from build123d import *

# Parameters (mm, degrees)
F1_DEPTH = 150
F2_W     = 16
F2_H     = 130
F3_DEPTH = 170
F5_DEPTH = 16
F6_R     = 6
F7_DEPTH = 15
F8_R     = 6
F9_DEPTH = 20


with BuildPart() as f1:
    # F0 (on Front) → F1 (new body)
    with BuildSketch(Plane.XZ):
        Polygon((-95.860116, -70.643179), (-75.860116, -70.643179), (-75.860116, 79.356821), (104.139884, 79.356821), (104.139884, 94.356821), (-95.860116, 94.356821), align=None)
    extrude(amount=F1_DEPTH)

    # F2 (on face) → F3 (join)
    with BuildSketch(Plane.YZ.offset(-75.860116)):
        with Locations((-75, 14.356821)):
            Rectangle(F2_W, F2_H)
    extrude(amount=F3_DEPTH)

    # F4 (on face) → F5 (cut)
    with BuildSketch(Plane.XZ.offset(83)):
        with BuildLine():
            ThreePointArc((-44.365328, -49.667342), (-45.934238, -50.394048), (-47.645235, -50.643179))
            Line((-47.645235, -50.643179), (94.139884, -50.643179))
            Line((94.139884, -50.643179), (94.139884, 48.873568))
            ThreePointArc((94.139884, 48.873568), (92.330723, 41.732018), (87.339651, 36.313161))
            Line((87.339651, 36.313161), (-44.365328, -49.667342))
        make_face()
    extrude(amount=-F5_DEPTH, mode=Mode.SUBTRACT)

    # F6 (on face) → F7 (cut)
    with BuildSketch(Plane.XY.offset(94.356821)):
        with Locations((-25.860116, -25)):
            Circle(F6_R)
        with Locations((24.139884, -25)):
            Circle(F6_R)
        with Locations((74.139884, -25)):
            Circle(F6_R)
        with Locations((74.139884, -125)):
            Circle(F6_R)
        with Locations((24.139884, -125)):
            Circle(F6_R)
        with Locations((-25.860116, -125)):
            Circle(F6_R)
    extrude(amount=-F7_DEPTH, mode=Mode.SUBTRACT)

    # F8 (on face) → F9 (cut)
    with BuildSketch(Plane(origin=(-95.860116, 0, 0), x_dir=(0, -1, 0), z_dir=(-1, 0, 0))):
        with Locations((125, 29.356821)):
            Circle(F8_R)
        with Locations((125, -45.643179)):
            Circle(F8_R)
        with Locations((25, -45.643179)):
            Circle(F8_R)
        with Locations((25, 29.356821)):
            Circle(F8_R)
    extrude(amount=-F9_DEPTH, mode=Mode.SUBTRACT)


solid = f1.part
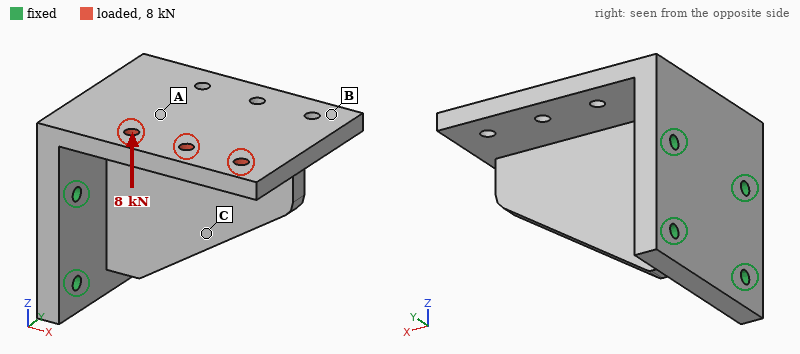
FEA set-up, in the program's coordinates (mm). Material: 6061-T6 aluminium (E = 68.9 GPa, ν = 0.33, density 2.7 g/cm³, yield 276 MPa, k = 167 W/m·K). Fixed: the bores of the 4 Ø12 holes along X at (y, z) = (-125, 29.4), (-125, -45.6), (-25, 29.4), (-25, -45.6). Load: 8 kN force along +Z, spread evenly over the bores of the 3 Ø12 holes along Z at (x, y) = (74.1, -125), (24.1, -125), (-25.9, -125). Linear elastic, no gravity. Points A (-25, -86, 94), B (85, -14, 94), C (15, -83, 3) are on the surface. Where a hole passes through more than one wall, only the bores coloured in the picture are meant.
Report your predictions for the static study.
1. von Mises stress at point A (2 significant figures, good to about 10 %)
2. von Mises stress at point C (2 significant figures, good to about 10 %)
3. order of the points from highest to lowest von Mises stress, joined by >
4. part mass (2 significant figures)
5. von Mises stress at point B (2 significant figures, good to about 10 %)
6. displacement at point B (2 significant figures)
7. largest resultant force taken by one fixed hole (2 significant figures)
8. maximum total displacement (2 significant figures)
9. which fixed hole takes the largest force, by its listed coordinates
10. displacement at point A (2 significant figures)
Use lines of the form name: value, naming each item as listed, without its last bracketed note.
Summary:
von Mises stress at point A: 35 MPa
von Mises stress at point C: 20 MPa
order of the points from highest to lowest von Mises stress, joined by >: A > C > B
part mass: 3.1 kg
von Mises stress at point B: 6.7 MPa
displacement at point B: 0.087 mm
largest resultant force taken by one fixed hole: 6.6 kN
maximum total displacement: 0.57 mm
which fixed hole takes the largest force, by its listed coordinates: (-125, 29.4)
displacement at point A: 0.097 mm
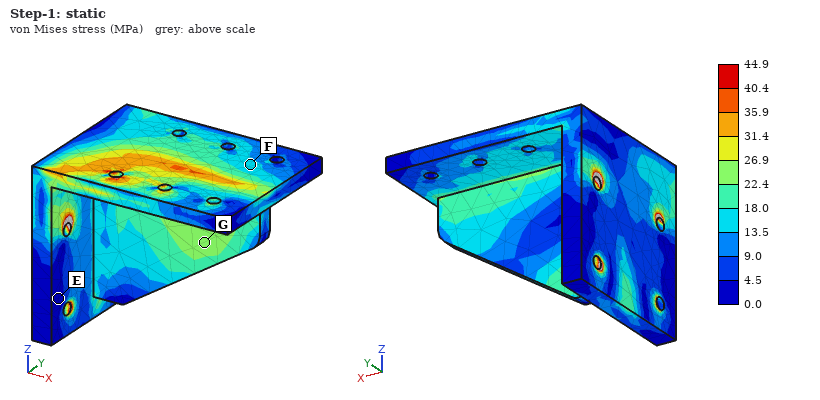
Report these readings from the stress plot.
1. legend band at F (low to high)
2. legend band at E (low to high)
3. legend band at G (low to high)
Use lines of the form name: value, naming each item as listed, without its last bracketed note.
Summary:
legend band at F: 13.5 to 18.0 MPa
legend band at E: 0.0 to 4.5 MPa
legend band at G: 22.4 to 26.9 MPa
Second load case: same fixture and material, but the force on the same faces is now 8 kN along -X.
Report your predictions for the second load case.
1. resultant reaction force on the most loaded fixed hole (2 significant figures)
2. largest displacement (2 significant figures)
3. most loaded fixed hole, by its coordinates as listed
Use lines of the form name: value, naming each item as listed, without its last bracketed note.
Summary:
resultant reaction force on the most loaded fixed hole: 9.7 kN
largest displacement: 0.21 mm
most loaded fixed hole, by its coordinates as listed: (-125, 29.4)
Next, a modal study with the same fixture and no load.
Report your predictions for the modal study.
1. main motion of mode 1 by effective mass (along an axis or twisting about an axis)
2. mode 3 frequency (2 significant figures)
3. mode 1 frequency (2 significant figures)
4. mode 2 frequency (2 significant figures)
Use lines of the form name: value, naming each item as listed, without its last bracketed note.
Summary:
main motion of mode 1 by effective mass: along Y
mode 3 frequency: 1200 Hz
mode 1 frequency: 790 Hz
mode 2 frequency: 1000 Hz
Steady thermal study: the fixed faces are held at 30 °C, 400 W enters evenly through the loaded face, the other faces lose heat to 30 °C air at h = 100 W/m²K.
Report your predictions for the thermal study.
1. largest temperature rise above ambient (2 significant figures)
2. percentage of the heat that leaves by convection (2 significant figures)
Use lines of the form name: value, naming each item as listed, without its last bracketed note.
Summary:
largest temperature rise above ambient: 72 K
percentage of the heat that leaves by convection: 69 %
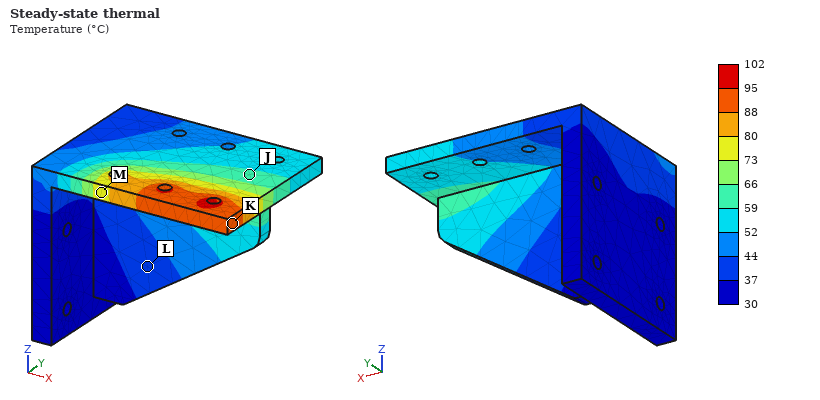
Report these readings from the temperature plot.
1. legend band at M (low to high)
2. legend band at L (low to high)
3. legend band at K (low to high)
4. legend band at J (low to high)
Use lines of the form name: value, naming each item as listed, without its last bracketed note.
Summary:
legend band at M: 73 to 80 °C
legend band at L: 37 to 44 °C
legend band at K: 88 to 95 °C
legend band at J: 59 to 66 °C
